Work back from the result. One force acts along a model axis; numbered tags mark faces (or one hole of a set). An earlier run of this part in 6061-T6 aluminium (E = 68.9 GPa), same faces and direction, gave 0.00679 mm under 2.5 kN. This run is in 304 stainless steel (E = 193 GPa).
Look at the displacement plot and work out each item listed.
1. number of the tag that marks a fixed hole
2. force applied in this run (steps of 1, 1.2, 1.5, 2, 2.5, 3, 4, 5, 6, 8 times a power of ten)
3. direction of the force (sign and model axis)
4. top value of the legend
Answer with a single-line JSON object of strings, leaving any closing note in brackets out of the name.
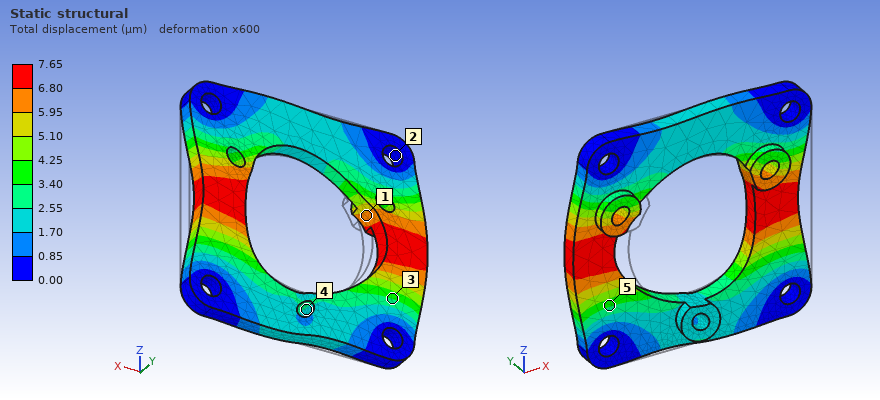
{"number of the tag that marks a fixed hole": "2", "force applied in this run": "8 kN", "direction of the force": "-X", "top value of the legend": "7.65 µm"}
